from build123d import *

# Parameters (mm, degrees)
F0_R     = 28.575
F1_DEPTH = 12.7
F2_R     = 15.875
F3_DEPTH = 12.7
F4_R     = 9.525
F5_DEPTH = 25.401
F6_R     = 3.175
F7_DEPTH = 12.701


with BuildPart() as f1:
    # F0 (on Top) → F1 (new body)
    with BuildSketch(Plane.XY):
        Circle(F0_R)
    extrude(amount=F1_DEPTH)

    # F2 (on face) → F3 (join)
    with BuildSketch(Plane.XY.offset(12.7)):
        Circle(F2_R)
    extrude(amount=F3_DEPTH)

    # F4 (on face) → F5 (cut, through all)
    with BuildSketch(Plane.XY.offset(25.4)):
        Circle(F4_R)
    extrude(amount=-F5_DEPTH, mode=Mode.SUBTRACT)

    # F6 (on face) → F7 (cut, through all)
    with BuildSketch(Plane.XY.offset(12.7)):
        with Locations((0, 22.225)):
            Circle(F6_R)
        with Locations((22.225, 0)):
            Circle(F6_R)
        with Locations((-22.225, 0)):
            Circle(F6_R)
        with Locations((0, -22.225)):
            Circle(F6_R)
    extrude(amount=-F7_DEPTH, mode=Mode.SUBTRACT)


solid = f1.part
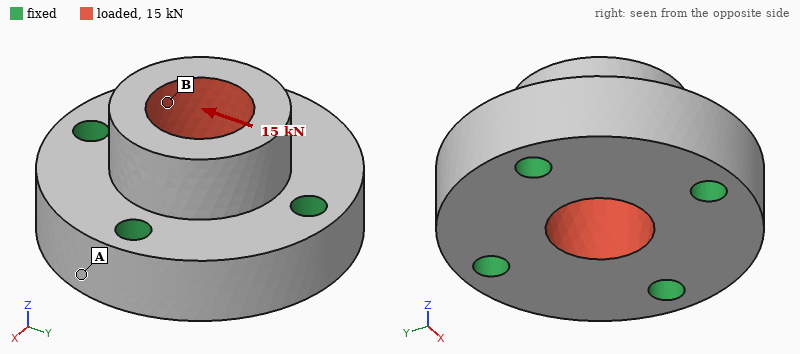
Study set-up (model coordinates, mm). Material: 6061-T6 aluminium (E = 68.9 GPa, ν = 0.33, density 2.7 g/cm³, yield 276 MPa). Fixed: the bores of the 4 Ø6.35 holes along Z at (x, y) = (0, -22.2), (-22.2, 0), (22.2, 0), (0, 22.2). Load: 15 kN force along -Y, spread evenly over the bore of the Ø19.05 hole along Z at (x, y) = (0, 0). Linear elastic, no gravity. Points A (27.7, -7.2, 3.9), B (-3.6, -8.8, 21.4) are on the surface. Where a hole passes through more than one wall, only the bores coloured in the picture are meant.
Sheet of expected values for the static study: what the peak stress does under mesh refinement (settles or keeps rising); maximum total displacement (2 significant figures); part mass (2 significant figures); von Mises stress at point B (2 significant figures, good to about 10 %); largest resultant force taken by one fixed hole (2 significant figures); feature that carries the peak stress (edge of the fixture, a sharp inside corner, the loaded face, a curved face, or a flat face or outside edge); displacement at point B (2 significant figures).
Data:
keeps rising
17 µm
91 g
21 MPa
4.9 kN
a sharp inside corner
13 µm
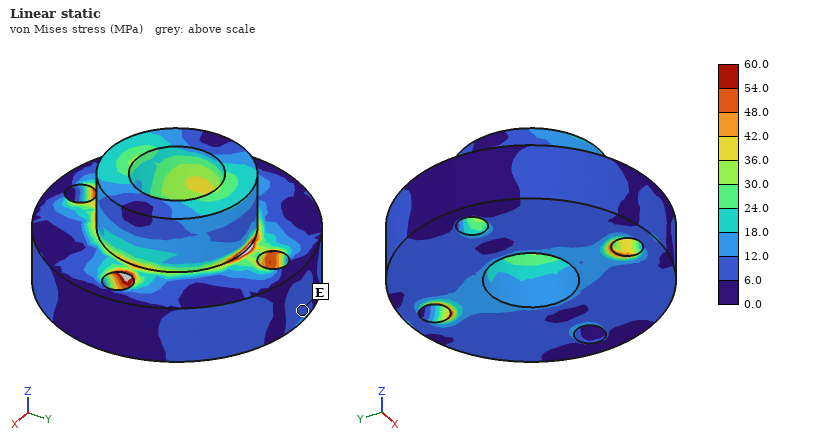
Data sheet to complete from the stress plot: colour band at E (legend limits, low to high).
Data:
6.0 to 12.0 MPa
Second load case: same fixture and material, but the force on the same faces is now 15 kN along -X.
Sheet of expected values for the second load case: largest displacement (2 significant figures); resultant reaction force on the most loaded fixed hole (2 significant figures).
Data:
17 µm
4.9 kN
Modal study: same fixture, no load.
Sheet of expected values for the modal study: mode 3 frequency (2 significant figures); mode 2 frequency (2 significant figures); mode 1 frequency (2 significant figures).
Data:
31 kHz
29 kHz
29 kHz
